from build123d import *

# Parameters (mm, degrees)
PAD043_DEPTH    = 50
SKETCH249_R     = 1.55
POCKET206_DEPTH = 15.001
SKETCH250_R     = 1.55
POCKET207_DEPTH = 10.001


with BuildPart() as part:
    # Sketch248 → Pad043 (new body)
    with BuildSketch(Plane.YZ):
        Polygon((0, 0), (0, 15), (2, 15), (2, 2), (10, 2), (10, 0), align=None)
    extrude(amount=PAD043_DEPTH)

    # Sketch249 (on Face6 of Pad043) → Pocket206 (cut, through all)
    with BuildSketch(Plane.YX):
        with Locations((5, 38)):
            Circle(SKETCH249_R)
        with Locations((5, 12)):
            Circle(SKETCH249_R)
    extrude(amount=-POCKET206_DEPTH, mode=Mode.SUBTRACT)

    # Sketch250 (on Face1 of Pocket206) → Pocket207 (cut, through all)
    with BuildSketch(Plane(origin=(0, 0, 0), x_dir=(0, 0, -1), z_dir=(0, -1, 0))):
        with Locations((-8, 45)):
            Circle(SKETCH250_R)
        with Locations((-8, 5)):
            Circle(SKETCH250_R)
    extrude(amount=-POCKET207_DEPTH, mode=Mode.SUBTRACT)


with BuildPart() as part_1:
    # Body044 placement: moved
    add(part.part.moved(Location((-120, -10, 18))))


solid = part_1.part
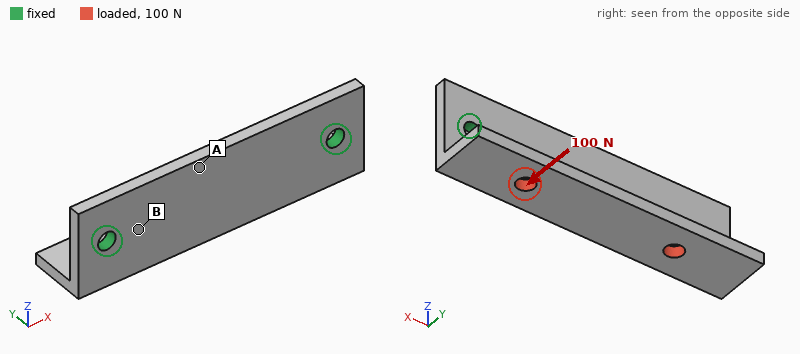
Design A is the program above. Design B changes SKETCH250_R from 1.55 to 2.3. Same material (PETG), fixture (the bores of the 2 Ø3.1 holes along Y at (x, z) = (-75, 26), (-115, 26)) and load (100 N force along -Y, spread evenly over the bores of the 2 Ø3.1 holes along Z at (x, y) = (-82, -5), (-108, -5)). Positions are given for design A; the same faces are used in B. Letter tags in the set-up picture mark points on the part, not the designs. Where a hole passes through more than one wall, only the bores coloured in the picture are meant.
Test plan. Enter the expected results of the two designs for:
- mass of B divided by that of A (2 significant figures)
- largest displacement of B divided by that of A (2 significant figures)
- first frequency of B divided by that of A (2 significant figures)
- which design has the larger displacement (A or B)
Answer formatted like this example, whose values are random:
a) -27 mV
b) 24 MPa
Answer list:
a) 0.98
b) 0.72
c) 1.1
d) A
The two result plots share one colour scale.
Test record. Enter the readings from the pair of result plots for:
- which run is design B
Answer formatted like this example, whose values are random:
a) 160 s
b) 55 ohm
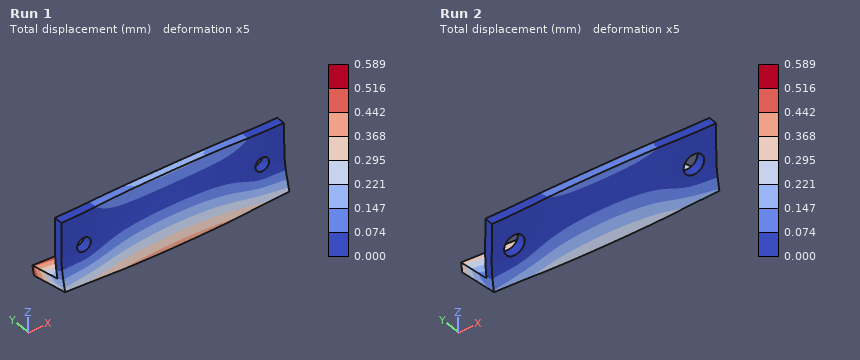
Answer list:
a) Run 2
